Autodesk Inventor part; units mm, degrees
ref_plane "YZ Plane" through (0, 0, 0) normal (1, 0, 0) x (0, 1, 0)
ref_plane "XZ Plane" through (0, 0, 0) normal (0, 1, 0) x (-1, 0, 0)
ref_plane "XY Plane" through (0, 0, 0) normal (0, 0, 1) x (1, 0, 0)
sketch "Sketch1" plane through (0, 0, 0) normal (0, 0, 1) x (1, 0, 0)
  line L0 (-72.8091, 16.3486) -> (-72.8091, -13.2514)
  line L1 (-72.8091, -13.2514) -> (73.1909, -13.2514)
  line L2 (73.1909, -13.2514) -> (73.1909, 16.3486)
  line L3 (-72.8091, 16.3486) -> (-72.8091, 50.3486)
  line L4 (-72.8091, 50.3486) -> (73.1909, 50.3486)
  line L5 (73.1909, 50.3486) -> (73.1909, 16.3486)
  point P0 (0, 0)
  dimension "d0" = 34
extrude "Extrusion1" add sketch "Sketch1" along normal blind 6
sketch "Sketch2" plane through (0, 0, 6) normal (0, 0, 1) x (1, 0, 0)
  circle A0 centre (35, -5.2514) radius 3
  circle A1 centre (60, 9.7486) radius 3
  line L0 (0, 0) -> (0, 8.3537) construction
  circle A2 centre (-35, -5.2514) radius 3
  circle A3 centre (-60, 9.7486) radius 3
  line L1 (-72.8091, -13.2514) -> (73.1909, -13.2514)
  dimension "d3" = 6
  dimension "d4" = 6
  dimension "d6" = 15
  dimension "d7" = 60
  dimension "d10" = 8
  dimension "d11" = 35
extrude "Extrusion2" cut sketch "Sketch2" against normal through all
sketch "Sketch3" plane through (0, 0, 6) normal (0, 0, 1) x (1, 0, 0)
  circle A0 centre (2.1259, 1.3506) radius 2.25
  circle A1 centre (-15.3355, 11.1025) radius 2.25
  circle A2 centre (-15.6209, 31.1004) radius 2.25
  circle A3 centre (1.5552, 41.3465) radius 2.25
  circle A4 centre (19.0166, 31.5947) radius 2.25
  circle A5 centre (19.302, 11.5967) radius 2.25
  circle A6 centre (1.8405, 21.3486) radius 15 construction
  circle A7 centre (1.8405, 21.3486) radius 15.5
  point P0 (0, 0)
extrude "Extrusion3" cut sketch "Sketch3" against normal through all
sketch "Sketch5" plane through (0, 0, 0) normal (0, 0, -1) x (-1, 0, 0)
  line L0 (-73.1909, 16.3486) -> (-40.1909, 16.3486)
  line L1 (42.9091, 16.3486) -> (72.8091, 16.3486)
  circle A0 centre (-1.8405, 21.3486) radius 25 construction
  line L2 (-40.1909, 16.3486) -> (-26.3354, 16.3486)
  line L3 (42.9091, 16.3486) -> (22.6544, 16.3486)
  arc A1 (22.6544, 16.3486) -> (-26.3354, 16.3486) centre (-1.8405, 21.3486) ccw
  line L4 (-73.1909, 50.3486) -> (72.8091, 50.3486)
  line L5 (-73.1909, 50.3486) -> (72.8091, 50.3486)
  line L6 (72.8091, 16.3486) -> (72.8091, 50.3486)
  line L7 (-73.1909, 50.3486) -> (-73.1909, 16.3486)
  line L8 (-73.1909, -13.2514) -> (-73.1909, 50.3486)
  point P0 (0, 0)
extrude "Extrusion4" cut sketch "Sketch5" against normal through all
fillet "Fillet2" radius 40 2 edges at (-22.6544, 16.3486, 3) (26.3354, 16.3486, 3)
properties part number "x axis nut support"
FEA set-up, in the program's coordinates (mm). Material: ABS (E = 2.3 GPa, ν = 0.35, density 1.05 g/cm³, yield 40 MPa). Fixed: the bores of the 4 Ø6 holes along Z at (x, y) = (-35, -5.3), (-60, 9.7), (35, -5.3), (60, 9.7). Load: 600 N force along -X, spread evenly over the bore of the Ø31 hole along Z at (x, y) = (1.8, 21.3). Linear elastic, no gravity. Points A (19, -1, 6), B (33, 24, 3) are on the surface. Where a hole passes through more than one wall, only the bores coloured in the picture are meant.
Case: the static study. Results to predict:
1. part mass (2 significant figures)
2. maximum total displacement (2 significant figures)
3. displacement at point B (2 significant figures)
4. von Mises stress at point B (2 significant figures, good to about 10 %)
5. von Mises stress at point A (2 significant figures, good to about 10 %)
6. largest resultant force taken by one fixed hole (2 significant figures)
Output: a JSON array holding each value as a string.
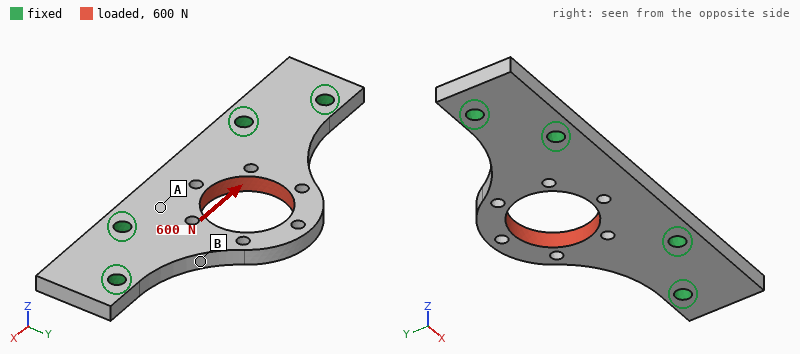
["31 g", "0.14 mm", "0.049 mm", "5.2 MPa", "1.1 MPa", "180 N"]
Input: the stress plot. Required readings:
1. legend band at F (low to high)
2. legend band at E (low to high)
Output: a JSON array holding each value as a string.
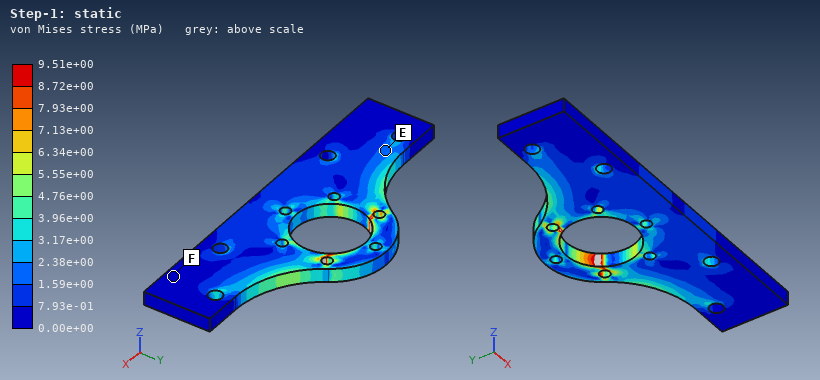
["0.00e+00 to 7.93e-01 MPa", "1.59e+00 to 2.38e+00 MPa"]
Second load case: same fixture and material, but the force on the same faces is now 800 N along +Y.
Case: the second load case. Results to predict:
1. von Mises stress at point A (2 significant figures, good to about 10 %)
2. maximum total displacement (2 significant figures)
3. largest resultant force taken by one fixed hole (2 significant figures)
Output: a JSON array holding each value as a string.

["2.7 MPa", "0.11 mm", "460 N"]
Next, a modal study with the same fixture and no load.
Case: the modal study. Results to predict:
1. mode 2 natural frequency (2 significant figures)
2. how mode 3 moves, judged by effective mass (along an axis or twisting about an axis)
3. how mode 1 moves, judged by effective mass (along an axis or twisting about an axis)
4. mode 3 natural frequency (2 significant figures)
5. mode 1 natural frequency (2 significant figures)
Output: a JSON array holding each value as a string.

["1800 Hz", "along Z", "along Z", "2000 Hz", "720 Hz"]
